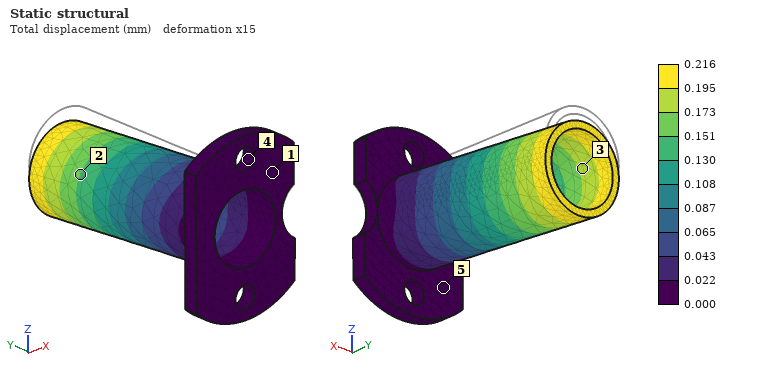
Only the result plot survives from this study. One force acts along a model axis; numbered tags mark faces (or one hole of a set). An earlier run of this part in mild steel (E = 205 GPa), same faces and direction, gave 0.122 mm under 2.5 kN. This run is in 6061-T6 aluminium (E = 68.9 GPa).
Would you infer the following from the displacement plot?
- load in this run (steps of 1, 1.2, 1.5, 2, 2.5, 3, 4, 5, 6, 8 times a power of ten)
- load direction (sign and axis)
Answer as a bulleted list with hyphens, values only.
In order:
- 1.5 kN
- -Z
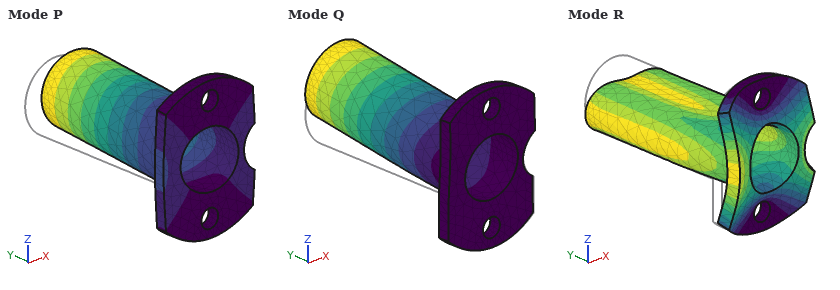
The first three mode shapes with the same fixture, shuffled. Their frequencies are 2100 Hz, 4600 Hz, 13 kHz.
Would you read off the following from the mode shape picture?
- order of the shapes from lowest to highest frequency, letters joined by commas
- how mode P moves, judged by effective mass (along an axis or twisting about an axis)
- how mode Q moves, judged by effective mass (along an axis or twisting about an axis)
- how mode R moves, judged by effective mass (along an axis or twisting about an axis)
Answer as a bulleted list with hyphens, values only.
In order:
- P, Q, R
- along X
- along Z
- along Y
